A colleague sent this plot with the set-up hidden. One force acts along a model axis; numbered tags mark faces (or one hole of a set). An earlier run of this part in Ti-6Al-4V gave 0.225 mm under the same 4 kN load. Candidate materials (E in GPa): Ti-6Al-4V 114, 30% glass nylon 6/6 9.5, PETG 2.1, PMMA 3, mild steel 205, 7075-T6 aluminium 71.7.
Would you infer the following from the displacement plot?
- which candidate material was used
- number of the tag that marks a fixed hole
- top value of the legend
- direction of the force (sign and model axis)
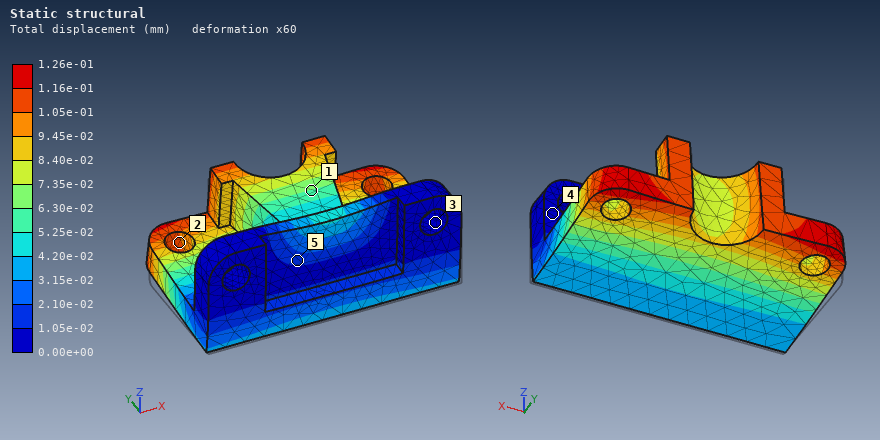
mild steel
3
1.26e-01 mm
+Z
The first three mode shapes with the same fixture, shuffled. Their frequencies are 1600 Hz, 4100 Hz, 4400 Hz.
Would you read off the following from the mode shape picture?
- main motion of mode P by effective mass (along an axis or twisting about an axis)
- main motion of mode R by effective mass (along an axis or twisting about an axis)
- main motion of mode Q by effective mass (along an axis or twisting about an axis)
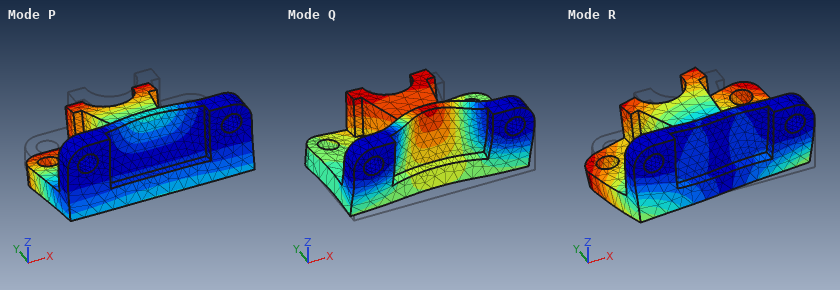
along Z
along X
along Y
